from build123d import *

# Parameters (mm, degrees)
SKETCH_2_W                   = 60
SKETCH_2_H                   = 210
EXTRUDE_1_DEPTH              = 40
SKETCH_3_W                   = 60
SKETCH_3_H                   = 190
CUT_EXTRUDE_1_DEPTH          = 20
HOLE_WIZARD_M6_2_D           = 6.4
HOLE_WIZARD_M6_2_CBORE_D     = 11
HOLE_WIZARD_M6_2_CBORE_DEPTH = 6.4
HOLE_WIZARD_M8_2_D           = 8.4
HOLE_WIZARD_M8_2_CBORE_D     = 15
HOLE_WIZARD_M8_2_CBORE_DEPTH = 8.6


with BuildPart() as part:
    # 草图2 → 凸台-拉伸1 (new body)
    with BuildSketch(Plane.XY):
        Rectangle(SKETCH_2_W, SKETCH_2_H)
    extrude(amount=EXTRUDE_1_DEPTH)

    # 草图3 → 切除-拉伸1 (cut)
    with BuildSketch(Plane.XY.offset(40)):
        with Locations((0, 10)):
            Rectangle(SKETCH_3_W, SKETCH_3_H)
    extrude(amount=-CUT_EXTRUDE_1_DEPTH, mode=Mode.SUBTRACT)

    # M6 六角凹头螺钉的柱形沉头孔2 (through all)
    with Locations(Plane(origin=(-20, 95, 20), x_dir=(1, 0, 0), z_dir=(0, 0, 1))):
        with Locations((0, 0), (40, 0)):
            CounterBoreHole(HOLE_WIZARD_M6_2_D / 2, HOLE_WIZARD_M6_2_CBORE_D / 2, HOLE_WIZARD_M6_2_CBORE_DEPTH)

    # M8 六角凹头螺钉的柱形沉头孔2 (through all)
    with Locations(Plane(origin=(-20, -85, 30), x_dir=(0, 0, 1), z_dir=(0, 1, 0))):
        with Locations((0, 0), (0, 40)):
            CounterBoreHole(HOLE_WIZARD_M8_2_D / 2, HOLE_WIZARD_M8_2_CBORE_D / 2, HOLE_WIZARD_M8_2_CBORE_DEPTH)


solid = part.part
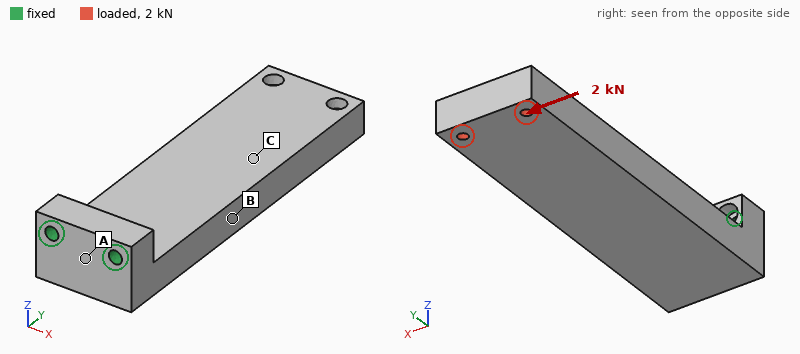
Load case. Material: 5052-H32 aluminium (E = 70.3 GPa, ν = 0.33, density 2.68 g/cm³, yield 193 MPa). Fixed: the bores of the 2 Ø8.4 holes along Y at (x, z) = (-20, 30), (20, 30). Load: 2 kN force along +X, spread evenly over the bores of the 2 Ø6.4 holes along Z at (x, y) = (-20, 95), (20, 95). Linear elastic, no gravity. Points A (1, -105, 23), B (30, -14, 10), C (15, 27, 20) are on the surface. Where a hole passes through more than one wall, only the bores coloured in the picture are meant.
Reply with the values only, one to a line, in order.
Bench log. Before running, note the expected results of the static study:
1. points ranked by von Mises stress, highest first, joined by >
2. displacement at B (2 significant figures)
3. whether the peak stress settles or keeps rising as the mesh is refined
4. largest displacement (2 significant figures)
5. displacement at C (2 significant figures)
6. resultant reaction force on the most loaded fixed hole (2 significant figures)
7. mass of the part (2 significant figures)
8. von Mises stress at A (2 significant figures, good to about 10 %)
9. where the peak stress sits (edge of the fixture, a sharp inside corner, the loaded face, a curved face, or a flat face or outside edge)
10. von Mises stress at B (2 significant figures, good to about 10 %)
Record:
A > B > C
0.15 mm
keeps rising
0.43 mm
0.23 mm
8.8 kN
720 g
32 MPa
edge of the fixture
18 MPa
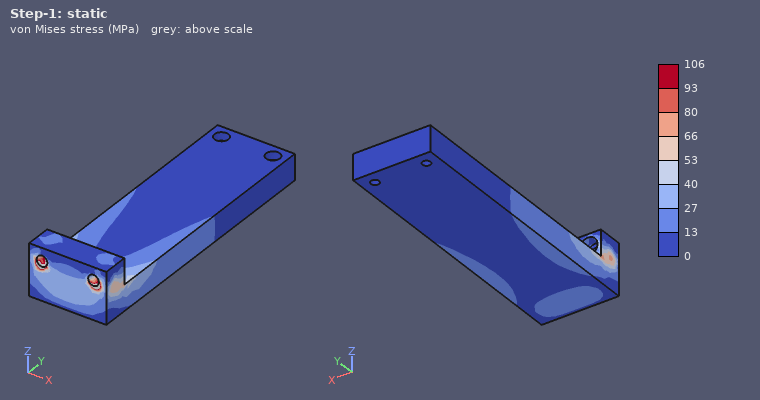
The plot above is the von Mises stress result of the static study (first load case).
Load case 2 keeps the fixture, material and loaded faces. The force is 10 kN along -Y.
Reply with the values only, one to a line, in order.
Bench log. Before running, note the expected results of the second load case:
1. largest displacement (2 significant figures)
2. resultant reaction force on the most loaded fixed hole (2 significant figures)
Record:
0.79 mm
5.0 kN
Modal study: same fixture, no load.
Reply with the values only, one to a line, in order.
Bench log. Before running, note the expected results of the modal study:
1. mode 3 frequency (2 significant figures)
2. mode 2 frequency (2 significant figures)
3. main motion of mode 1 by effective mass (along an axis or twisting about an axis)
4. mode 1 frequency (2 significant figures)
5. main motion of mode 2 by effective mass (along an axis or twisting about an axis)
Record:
2000 Hz
780 Hz
along Z
310 Hz
along X
